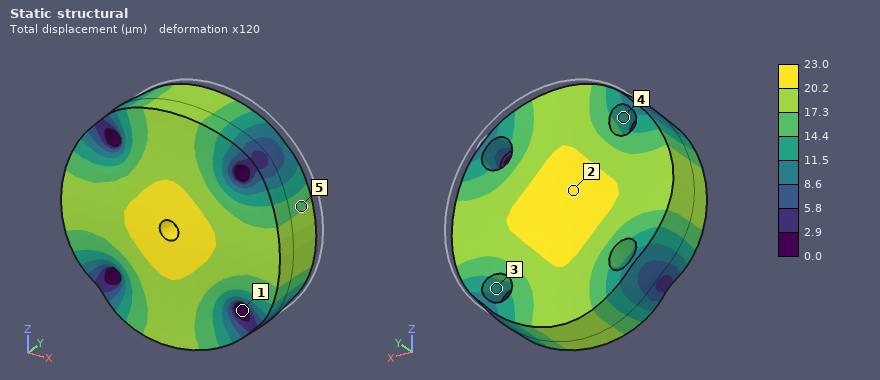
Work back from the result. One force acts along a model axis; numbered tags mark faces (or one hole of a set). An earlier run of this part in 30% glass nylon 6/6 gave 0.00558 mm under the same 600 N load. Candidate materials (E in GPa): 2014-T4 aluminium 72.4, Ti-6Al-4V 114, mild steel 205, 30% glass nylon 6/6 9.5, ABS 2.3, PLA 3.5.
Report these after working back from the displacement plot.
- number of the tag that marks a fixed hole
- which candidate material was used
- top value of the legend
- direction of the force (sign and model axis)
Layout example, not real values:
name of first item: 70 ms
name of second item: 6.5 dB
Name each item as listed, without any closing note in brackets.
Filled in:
number of the tag that marks a fixed hole: 1
which candidate material was used: ABS
top value of the legend: 23.0 µm
direction of the force: -Y
